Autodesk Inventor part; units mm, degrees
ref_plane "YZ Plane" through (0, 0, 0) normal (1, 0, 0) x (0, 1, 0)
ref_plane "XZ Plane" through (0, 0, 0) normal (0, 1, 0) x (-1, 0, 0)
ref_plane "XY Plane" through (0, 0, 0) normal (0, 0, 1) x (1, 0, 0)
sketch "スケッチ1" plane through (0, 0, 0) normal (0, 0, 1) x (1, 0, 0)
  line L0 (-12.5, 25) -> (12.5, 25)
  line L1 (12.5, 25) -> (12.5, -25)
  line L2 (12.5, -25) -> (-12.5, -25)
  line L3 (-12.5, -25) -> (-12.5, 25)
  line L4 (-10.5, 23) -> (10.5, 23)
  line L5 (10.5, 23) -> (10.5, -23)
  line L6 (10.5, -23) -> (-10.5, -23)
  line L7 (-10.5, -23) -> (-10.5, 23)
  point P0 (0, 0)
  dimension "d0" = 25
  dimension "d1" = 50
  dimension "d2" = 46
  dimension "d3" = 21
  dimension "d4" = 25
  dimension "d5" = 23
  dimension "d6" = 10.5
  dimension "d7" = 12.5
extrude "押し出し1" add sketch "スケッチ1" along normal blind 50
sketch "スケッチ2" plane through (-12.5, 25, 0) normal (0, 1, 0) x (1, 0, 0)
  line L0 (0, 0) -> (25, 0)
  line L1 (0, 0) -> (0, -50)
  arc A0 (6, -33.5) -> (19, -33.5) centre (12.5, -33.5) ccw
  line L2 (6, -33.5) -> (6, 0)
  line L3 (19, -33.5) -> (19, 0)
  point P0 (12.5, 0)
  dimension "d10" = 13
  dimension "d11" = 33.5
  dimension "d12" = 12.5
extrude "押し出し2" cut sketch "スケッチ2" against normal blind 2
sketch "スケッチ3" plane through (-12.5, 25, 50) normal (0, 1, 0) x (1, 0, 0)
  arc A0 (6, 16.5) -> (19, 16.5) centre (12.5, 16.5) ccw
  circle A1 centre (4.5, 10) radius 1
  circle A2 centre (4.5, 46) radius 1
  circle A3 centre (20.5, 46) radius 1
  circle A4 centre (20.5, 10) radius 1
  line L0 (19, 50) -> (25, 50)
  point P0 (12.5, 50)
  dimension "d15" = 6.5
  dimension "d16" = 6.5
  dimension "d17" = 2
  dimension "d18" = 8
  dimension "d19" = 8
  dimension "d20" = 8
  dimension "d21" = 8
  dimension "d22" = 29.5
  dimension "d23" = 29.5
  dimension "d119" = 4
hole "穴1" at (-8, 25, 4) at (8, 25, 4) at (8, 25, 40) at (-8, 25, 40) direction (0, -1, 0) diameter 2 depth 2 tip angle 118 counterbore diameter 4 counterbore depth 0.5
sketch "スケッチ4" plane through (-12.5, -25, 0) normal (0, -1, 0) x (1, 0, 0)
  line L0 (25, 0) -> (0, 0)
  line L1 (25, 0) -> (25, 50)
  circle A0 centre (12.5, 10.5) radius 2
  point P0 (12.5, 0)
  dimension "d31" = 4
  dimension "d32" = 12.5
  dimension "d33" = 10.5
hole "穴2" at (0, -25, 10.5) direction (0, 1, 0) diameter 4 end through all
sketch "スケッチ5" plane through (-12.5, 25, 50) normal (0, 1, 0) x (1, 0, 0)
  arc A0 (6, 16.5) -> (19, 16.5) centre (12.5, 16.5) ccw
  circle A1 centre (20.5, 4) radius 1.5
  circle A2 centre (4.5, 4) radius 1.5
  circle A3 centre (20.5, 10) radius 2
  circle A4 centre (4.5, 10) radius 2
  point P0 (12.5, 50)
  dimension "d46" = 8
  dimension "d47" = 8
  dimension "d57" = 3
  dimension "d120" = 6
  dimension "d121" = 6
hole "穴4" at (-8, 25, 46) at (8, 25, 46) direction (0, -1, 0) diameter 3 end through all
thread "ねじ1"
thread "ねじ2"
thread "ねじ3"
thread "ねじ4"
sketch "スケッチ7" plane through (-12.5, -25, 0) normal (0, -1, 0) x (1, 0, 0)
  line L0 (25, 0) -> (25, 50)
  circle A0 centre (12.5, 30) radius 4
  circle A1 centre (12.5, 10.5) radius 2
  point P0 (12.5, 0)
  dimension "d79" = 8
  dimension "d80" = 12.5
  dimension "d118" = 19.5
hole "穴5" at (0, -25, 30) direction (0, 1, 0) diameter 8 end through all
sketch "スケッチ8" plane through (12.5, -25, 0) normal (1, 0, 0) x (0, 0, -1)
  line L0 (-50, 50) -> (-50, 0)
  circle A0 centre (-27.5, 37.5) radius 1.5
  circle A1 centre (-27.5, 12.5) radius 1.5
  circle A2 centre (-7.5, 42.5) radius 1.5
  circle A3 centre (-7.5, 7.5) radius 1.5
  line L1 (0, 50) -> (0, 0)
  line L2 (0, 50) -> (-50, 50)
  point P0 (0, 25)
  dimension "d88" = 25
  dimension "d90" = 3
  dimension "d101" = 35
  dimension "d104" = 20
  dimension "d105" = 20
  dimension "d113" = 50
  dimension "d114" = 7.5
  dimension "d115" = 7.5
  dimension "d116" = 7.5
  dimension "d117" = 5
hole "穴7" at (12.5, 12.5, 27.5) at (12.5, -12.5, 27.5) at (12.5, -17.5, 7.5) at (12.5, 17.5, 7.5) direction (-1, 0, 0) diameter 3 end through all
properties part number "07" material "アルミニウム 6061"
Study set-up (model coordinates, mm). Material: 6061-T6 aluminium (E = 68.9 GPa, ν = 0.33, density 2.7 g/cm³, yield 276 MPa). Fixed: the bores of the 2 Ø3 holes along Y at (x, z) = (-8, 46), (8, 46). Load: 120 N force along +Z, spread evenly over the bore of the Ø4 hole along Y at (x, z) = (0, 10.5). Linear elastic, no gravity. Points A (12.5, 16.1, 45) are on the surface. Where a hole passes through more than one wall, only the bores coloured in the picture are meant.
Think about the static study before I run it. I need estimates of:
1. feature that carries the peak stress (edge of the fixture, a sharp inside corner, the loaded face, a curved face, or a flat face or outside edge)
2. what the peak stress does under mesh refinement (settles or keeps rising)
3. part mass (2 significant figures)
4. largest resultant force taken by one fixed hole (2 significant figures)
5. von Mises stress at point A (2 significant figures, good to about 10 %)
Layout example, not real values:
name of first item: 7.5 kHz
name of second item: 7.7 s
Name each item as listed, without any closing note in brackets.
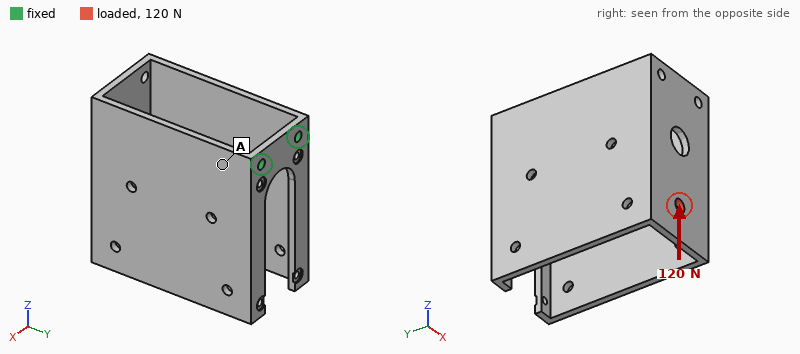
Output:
feature that carries the peak stress: edge of the fixture
what the peak stress does under mesh refinement: keeps rising
part mass: 35 g
largest resultant force taken by one fixed hole: 61 N
von Mises stress at point A: 26 MPa
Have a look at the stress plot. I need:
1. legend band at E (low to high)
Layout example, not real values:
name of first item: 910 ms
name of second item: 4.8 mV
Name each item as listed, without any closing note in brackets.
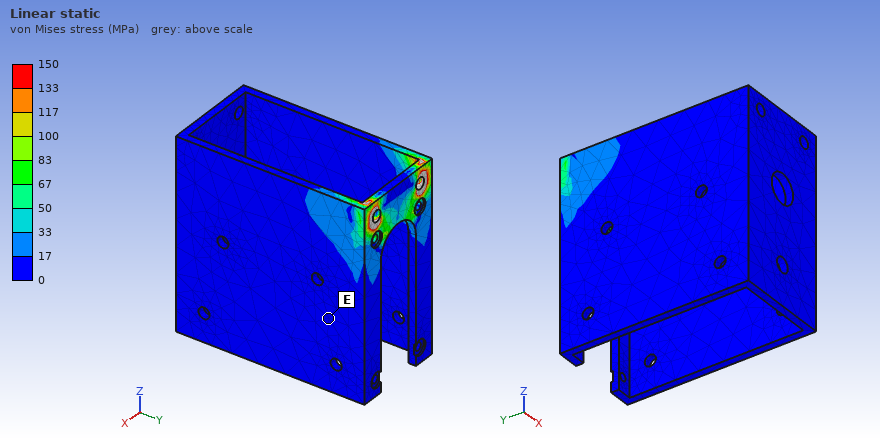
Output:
legend band at E: 0 to 17 MPa
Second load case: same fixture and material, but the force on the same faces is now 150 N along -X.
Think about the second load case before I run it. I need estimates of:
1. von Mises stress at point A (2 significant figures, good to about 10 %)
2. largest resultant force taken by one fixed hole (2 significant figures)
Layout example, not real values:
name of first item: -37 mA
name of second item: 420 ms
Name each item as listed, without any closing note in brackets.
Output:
von Mises stress at point A: 60 MPa
largest resultant force taken by one fixed hole: 360 N
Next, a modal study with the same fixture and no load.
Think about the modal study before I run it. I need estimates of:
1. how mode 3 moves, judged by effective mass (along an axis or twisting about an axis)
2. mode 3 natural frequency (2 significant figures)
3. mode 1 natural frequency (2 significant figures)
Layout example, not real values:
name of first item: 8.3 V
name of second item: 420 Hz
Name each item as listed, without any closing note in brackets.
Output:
how mode 3 moves, judged by effective mass: twisting about Y
mode 3 natural frequency: 1100 Hz
mode 1 natural frequency: 560 Hz
